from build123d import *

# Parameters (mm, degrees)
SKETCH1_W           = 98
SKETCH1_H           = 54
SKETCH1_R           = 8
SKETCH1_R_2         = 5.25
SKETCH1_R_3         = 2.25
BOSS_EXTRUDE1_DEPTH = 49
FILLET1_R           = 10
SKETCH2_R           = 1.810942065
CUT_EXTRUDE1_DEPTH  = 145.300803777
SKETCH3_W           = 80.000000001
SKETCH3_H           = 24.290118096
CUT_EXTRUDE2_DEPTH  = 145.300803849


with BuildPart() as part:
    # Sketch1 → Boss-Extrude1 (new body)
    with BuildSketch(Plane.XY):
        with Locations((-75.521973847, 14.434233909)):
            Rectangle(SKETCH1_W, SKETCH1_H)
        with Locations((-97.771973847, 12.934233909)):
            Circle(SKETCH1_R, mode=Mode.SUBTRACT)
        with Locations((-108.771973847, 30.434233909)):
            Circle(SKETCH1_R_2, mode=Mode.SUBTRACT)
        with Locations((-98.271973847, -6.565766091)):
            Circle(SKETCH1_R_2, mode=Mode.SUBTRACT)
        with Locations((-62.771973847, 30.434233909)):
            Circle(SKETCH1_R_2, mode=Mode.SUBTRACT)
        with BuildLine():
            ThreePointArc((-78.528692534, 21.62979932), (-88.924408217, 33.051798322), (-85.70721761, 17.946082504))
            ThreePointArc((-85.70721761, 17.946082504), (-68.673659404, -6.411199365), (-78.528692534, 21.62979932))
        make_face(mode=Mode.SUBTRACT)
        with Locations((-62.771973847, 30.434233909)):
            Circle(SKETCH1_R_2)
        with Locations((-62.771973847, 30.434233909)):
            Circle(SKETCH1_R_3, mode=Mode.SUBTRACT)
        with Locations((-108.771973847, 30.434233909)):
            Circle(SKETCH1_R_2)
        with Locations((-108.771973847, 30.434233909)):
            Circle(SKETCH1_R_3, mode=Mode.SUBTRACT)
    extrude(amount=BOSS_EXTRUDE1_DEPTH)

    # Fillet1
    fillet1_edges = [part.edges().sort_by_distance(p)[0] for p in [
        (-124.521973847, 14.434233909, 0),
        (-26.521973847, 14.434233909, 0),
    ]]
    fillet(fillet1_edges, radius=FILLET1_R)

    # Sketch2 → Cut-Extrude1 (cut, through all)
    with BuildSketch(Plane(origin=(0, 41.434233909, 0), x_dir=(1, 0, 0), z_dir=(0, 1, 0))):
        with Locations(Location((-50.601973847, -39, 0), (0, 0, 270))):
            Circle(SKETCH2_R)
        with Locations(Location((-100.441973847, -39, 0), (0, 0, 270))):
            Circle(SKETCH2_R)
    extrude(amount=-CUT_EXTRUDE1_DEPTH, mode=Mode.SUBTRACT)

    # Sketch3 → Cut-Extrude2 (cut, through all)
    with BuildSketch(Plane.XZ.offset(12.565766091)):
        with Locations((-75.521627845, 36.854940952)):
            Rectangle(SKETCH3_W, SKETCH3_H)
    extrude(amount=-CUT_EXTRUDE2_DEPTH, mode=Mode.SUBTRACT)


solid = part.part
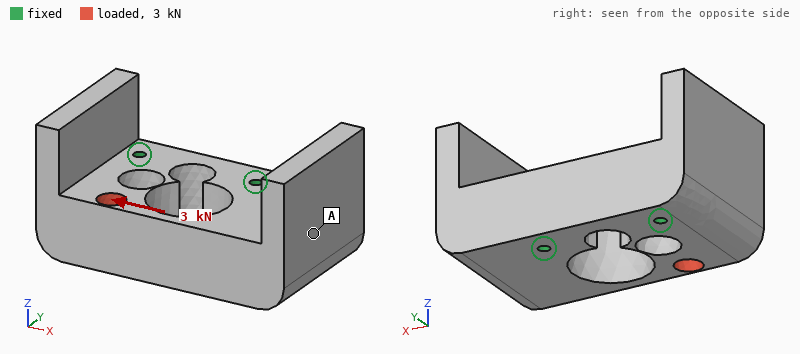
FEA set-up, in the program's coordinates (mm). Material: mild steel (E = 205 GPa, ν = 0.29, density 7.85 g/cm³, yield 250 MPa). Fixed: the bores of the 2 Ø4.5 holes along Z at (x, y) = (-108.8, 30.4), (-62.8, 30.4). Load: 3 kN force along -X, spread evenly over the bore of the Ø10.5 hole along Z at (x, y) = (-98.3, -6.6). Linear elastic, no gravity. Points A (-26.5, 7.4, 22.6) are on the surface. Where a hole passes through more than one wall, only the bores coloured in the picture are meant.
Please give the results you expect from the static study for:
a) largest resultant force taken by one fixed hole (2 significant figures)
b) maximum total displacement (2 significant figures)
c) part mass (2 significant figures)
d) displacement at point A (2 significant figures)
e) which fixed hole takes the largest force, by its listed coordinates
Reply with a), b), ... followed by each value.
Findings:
a) 2.6 kN
b) 12 µm
c) 960 g
d) 8.2 µm
e) (-108.8, 30.4)
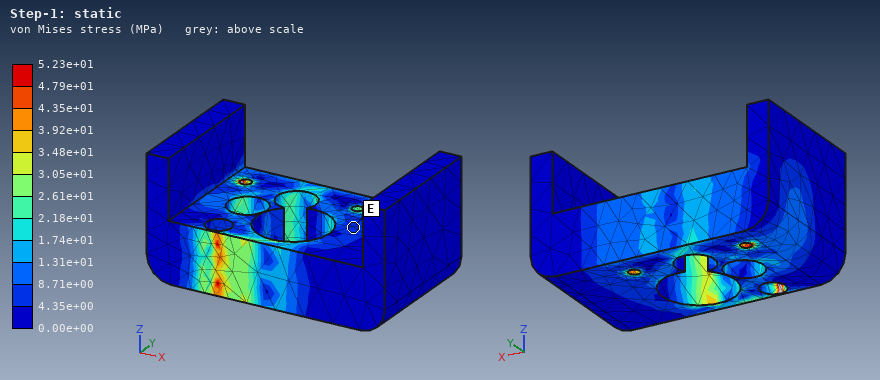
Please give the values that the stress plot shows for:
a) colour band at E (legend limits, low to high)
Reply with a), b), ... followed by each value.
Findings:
a) 4.35e+00 to 8.71e+00 MPa
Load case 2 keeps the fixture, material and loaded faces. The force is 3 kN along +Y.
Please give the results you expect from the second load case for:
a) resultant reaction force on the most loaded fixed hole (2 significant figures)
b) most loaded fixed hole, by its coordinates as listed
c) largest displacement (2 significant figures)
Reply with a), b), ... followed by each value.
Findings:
a) 2.5 kN
b) (-108.8, 30.4)
c) 6.4 µm
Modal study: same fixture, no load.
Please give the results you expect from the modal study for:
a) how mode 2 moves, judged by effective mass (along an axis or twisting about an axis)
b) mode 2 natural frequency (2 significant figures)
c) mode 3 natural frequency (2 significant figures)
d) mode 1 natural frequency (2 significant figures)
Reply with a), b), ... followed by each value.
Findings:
a) along Z
b) 4300 Hz
c) 5700 Hz
d) 3900 Hz
